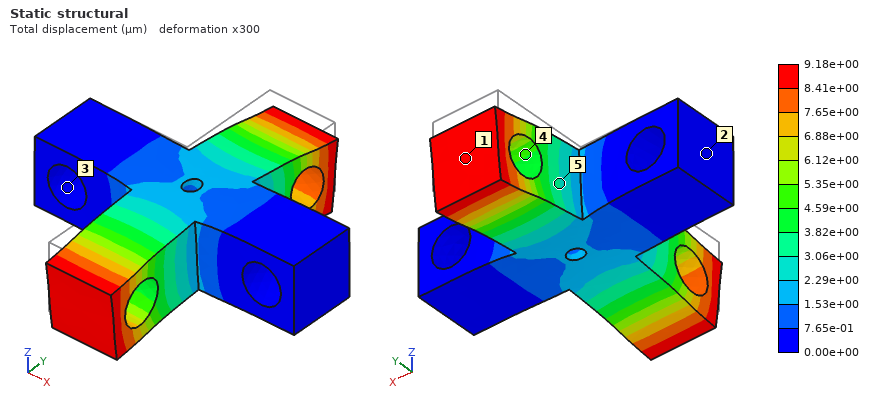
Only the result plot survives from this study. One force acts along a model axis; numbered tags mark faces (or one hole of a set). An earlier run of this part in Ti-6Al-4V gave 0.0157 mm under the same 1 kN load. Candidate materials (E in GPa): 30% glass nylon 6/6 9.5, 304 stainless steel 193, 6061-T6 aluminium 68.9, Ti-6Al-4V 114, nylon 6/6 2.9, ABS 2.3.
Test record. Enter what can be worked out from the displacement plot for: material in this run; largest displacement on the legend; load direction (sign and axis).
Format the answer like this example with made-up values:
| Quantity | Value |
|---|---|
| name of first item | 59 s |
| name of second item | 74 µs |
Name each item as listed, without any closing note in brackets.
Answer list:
| Quantity | Value |
|---|---|
| material in this run | 304 stainless steel |
| largest displacement on the legend | 9.18e+00 µm |
| load direction | -Z |
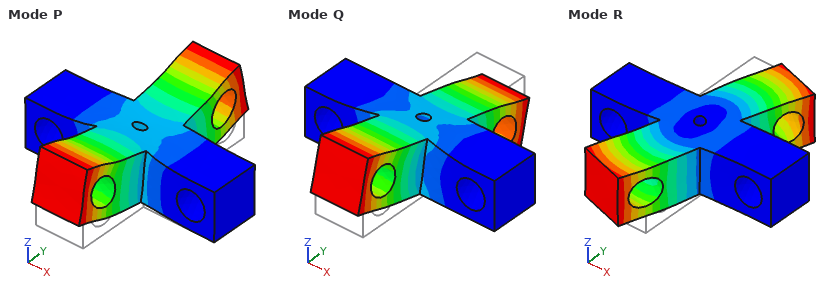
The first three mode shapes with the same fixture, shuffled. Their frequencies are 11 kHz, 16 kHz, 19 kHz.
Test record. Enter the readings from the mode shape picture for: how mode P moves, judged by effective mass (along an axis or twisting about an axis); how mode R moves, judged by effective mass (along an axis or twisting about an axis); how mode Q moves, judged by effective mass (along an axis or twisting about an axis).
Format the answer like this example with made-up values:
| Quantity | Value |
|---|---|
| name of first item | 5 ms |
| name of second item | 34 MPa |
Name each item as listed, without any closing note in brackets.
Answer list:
| Quantity | Value |
|---|---|
| how mode P moves, judged by effective mass | along Z |
| how mode R moves, judged by effective mass | twisting about Z |
| how mode Q moves, judged by effective mass | twisting about X |
